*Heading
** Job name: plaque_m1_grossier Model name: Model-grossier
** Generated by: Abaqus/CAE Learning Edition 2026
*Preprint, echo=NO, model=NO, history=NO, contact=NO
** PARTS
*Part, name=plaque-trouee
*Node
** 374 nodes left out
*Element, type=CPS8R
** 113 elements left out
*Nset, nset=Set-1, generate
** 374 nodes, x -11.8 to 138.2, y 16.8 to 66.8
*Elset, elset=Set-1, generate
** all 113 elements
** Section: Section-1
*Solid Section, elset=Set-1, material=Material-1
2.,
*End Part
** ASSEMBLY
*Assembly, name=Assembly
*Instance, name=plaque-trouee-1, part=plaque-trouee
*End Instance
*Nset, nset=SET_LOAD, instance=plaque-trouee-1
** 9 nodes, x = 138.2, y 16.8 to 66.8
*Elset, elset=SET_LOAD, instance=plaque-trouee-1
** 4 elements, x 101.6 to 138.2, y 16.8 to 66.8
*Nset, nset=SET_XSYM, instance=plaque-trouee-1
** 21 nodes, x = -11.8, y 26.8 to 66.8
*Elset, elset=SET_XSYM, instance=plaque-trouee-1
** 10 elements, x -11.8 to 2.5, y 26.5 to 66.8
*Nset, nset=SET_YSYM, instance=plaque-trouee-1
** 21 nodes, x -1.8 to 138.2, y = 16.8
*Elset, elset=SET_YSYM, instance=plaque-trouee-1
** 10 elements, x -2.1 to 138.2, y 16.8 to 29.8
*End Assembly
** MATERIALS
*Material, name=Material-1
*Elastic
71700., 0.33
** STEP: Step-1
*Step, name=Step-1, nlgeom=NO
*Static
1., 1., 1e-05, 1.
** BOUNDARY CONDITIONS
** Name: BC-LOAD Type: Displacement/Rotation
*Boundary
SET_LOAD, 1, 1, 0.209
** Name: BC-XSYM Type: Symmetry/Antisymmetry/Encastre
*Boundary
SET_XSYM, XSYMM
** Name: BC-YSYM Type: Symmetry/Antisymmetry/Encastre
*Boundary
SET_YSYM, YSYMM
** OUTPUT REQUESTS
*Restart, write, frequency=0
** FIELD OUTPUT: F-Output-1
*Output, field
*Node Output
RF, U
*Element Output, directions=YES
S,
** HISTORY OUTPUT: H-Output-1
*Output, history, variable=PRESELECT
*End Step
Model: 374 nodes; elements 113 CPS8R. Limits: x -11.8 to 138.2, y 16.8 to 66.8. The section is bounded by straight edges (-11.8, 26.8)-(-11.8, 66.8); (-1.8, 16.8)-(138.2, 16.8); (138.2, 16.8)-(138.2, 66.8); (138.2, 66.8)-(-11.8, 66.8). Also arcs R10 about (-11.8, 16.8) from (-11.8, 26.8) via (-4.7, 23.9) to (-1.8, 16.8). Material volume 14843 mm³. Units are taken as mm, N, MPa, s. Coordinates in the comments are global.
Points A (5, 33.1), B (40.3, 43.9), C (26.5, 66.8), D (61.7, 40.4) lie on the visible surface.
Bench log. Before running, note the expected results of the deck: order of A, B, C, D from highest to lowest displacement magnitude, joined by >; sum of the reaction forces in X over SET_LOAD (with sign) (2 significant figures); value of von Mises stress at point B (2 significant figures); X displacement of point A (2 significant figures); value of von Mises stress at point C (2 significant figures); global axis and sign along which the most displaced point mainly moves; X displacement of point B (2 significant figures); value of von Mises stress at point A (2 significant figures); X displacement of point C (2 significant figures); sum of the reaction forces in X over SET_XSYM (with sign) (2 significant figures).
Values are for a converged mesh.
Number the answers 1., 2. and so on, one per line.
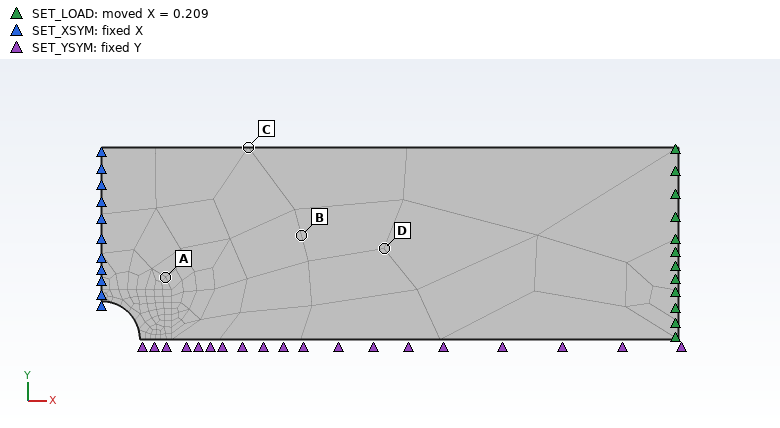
1. D > B > C > A
2. 9700 N
3. 98 MPa
4. 0.030 mm
5. 110 MPa
6. +X
7. 0.077 mm
8. 120 MPa
9. 0.054 mm
10. -9700 N
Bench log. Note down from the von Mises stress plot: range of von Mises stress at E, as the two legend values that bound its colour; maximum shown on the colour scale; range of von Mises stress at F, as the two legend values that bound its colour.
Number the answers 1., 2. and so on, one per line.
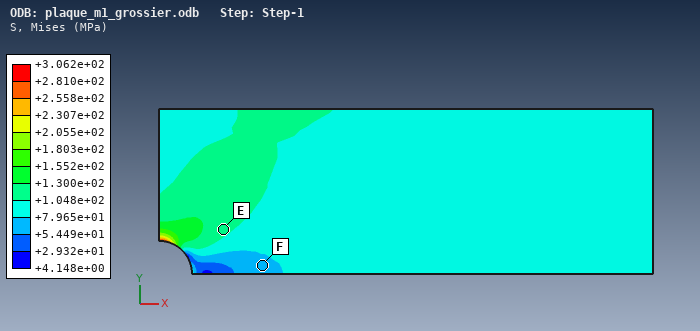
1. +1.048e+02 to +1.300e+02 MPa
2. +3.062e+02 MPa
3. +5.449e+01 to +7.965e+01 MPa
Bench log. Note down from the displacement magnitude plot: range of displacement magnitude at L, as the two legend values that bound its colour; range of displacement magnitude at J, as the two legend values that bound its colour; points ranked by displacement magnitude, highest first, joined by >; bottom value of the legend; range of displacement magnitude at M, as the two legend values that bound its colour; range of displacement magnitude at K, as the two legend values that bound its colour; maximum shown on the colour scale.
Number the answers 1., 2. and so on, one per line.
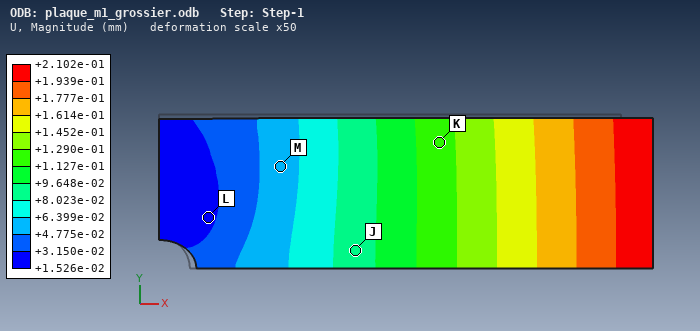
1. +1.526e-02 to +3.150e-02 mm
2. +8.023e-02 to +9.648e-02 mm
3. K > J > M > L
4. +1.526e-02 mm
5. +4.775e-02 to +6.399e-02 mm
6. +1.127e-01 to +1.290e-01 mm
7. +2.102e-01 mm
